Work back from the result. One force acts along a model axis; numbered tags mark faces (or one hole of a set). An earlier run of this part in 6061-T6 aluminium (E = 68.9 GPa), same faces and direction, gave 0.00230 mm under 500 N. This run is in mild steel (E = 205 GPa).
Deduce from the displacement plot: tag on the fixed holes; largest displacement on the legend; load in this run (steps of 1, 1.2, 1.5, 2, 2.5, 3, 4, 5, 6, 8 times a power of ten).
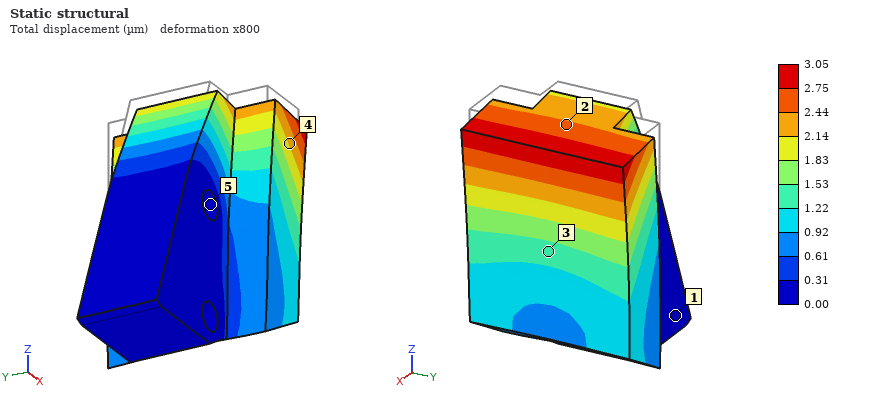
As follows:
5
3.05 µm
2 kN
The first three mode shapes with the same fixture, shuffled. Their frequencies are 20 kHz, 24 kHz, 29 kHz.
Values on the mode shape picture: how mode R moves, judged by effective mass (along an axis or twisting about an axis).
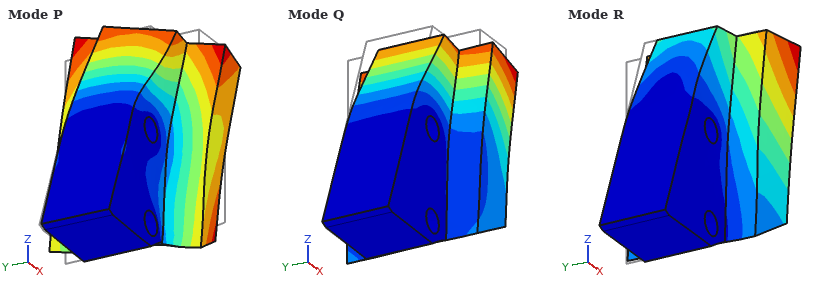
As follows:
along Y
